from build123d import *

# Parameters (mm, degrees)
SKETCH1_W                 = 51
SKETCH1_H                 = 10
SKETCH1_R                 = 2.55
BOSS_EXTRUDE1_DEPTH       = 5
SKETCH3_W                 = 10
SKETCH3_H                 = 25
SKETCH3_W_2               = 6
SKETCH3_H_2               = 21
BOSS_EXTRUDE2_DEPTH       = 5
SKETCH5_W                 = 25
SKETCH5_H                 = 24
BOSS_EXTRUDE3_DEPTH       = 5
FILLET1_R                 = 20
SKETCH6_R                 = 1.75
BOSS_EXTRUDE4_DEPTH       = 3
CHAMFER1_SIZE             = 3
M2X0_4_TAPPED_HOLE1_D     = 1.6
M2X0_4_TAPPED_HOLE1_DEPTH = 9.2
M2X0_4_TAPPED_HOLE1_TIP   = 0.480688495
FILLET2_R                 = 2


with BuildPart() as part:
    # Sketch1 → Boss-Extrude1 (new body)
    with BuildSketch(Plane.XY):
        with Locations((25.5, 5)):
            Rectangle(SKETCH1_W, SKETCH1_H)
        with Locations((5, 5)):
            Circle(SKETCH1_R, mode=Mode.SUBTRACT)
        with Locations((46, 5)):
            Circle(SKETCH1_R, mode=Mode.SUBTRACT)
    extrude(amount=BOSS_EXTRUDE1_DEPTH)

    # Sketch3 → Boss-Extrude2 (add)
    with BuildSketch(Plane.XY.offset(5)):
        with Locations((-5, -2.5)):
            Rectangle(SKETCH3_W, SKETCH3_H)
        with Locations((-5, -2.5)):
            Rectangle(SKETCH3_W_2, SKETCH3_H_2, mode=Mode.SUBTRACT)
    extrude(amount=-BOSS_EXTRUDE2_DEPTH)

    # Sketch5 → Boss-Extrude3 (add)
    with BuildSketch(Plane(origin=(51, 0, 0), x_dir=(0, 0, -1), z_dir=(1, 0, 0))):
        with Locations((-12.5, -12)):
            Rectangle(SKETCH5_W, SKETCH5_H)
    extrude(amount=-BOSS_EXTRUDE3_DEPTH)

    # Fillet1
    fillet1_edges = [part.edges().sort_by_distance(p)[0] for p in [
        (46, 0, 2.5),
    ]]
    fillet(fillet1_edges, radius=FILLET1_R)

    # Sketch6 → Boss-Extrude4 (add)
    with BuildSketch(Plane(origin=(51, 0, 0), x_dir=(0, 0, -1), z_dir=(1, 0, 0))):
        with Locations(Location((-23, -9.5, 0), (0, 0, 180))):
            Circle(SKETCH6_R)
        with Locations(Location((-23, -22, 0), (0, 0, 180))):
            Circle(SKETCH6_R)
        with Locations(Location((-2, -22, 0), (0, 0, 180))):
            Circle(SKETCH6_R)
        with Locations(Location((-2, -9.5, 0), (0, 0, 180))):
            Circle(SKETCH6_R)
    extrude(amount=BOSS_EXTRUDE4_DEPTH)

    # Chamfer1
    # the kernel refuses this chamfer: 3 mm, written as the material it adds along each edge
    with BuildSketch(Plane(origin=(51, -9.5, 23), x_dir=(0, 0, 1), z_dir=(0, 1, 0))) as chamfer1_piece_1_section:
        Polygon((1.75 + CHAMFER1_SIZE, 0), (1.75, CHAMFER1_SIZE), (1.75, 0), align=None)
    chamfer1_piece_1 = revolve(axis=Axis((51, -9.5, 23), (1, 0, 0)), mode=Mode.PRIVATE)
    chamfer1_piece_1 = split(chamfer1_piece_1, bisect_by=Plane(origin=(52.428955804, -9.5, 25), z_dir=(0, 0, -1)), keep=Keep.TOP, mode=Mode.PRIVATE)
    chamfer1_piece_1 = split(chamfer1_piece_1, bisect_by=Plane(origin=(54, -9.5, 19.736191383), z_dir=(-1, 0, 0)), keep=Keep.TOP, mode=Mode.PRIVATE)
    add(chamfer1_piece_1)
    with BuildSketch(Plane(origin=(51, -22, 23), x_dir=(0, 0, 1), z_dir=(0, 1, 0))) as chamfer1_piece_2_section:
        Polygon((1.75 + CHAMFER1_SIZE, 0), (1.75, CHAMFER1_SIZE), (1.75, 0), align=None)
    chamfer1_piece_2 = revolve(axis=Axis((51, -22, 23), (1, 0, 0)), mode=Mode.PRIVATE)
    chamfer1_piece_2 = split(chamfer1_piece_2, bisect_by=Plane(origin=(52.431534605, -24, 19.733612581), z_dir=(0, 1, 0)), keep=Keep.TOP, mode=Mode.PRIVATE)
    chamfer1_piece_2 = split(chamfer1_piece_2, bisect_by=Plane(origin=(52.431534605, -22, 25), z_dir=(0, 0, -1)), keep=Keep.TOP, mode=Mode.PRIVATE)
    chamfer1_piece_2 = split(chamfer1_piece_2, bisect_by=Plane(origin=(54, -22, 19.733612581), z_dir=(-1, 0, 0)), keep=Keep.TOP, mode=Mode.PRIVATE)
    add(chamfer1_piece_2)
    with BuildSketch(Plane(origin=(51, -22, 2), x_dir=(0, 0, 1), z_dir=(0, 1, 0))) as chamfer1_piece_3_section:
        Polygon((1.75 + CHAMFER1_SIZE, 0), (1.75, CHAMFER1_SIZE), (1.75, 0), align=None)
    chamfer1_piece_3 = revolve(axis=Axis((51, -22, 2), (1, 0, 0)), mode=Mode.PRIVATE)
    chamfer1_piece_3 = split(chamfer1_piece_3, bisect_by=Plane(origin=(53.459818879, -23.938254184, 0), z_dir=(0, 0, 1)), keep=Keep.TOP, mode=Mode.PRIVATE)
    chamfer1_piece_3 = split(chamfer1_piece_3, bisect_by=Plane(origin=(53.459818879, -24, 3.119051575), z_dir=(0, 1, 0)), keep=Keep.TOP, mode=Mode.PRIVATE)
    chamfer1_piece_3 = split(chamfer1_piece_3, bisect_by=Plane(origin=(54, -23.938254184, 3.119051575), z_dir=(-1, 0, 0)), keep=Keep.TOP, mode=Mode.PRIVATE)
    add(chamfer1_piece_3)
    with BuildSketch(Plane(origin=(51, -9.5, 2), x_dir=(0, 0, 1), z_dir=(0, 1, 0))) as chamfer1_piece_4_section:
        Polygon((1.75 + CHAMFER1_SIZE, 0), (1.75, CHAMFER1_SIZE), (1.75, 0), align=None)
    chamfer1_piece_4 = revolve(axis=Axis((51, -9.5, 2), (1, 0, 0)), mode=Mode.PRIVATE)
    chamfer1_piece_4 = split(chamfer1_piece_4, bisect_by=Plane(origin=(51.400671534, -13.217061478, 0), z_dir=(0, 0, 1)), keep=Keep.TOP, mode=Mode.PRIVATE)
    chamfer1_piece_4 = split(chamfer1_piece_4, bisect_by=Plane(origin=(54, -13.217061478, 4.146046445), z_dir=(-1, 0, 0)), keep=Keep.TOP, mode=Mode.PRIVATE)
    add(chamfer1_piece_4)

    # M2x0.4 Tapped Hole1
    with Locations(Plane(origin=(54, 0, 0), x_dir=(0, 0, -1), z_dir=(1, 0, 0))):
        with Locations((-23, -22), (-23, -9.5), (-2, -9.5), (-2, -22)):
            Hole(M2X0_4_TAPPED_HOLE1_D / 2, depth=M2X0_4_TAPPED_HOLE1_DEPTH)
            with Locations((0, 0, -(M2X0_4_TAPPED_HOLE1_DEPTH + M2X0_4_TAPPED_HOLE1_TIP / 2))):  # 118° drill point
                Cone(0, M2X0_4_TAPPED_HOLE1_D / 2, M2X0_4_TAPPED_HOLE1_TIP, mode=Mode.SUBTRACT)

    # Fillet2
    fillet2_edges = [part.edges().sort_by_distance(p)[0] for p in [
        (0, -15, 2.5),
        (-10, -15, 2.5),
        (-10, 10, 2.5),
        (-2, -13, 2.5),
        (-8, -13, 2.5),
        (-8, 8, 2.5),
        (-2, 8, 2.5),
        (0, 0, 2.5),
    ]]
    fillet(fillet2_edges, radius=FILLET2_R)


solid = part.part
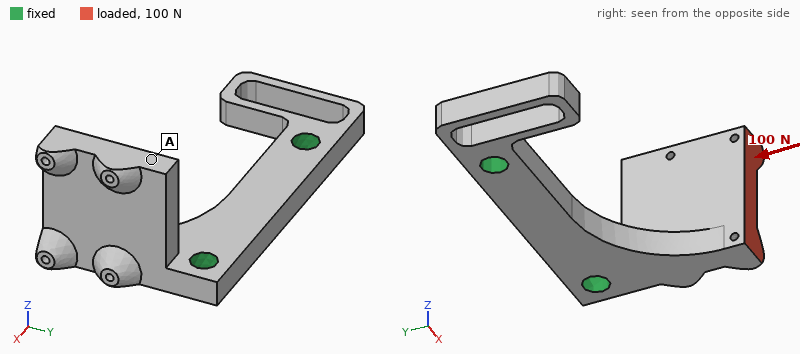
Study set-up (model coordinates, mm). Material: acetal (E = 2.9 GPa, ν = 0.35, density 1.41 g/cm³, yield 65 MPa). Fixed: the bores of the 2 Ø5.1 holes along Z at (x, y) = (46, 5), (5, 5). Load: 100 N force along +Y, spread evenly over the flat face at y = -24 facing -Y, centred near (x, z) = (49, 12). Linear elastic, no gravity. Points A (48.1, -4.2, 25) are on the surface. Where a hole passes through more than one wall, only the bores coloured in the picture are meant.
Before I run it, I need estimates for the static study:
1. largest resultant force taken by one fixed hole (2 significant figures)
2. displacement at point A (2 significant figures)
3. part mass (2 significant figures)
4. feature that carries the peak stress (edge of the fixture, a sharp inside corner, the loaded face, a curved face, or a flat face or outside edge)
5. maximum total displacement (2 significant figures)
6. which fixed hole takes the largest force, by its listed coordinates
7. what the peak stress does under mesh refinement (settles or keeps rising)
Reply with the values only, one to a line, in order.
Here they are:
100 N
0.46 mm
9.4 g
edge of the fixture
0.67 mm
(46, 5)
keeps rising
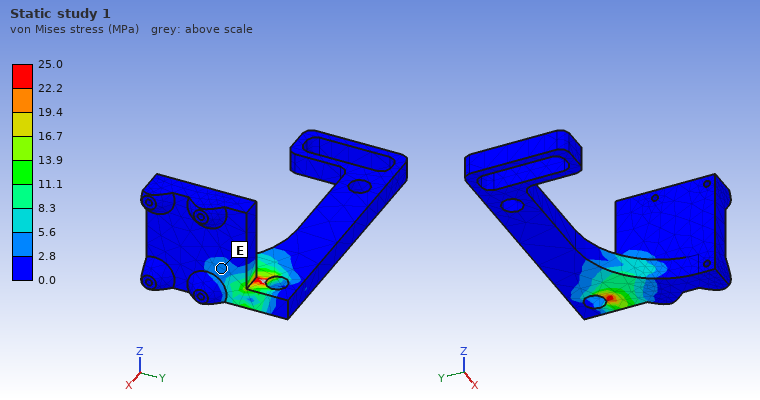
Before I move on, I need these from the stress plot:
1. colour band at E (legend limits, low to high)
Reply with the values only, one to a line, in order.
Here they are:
2.8 to 5.6 MPa
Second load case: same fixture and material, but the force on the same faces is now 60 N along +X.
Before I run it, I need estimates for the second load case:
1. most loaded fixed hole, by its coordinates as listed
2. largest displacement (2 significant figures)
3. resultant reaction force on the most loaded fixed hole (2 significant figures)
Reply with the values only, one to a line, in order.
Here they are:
(46, 5)
0.79 mm
42 N
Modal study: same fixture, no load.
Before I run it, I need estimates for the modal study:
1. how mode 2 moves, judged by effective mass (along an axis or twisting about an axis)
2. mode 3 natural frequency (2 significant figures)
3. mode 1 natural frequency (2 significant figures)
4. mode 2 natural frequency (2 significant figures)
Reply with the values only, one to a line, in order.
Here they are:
along X
1400 Hz
850 Hz
1100 Hz
